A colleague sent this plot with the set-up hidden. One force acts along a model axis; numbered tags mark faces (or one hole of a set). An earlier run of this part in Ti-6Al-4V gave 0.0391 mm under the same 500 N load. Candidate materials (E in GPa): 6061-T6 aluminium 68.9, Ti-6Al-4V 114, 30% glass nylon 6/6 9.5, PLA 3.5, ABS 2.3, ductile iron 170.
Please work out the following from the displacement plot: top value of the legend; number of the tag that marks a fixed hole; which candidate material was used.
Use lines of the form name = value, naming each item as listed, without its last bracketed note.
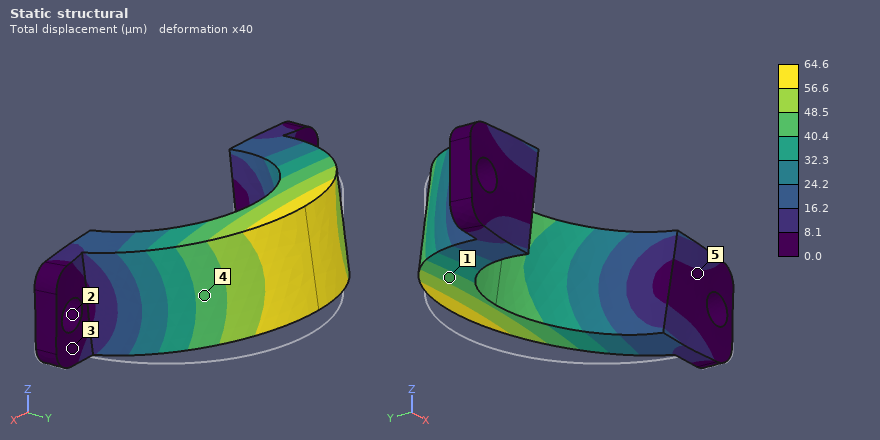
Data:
top value of the legend = 64.6 µm
number of the tag that marks a fixed hole = 2
which candidate material was used = 6061-T6 aluminium
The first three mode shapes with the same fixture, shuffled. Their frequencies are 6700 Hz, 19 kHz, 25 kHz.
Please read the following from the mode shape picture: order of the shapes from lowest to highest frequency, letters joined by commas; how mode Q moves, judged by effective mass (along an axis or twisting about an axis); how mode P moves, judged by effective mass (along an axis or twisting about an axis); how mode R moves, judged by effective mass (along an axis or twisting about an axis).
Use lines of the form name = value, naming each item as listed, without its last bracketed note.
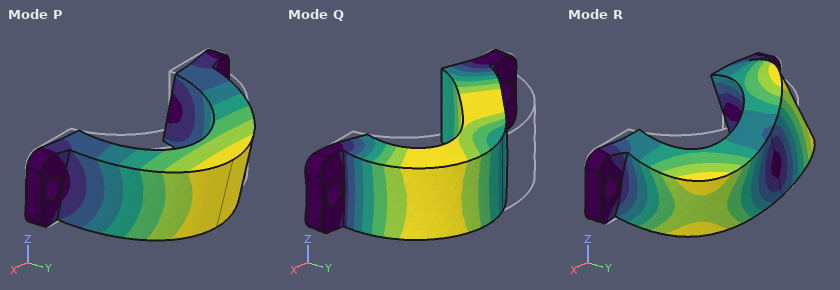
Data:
order of the shapes from lowest to highest frequency, letters joined by commas = P, Q, R
how mode Q moves, judged by effective mass = along X
how mode P moves, judged by effective mass = along Z
how mode R moves, judged by effective mass = twisting about Y
